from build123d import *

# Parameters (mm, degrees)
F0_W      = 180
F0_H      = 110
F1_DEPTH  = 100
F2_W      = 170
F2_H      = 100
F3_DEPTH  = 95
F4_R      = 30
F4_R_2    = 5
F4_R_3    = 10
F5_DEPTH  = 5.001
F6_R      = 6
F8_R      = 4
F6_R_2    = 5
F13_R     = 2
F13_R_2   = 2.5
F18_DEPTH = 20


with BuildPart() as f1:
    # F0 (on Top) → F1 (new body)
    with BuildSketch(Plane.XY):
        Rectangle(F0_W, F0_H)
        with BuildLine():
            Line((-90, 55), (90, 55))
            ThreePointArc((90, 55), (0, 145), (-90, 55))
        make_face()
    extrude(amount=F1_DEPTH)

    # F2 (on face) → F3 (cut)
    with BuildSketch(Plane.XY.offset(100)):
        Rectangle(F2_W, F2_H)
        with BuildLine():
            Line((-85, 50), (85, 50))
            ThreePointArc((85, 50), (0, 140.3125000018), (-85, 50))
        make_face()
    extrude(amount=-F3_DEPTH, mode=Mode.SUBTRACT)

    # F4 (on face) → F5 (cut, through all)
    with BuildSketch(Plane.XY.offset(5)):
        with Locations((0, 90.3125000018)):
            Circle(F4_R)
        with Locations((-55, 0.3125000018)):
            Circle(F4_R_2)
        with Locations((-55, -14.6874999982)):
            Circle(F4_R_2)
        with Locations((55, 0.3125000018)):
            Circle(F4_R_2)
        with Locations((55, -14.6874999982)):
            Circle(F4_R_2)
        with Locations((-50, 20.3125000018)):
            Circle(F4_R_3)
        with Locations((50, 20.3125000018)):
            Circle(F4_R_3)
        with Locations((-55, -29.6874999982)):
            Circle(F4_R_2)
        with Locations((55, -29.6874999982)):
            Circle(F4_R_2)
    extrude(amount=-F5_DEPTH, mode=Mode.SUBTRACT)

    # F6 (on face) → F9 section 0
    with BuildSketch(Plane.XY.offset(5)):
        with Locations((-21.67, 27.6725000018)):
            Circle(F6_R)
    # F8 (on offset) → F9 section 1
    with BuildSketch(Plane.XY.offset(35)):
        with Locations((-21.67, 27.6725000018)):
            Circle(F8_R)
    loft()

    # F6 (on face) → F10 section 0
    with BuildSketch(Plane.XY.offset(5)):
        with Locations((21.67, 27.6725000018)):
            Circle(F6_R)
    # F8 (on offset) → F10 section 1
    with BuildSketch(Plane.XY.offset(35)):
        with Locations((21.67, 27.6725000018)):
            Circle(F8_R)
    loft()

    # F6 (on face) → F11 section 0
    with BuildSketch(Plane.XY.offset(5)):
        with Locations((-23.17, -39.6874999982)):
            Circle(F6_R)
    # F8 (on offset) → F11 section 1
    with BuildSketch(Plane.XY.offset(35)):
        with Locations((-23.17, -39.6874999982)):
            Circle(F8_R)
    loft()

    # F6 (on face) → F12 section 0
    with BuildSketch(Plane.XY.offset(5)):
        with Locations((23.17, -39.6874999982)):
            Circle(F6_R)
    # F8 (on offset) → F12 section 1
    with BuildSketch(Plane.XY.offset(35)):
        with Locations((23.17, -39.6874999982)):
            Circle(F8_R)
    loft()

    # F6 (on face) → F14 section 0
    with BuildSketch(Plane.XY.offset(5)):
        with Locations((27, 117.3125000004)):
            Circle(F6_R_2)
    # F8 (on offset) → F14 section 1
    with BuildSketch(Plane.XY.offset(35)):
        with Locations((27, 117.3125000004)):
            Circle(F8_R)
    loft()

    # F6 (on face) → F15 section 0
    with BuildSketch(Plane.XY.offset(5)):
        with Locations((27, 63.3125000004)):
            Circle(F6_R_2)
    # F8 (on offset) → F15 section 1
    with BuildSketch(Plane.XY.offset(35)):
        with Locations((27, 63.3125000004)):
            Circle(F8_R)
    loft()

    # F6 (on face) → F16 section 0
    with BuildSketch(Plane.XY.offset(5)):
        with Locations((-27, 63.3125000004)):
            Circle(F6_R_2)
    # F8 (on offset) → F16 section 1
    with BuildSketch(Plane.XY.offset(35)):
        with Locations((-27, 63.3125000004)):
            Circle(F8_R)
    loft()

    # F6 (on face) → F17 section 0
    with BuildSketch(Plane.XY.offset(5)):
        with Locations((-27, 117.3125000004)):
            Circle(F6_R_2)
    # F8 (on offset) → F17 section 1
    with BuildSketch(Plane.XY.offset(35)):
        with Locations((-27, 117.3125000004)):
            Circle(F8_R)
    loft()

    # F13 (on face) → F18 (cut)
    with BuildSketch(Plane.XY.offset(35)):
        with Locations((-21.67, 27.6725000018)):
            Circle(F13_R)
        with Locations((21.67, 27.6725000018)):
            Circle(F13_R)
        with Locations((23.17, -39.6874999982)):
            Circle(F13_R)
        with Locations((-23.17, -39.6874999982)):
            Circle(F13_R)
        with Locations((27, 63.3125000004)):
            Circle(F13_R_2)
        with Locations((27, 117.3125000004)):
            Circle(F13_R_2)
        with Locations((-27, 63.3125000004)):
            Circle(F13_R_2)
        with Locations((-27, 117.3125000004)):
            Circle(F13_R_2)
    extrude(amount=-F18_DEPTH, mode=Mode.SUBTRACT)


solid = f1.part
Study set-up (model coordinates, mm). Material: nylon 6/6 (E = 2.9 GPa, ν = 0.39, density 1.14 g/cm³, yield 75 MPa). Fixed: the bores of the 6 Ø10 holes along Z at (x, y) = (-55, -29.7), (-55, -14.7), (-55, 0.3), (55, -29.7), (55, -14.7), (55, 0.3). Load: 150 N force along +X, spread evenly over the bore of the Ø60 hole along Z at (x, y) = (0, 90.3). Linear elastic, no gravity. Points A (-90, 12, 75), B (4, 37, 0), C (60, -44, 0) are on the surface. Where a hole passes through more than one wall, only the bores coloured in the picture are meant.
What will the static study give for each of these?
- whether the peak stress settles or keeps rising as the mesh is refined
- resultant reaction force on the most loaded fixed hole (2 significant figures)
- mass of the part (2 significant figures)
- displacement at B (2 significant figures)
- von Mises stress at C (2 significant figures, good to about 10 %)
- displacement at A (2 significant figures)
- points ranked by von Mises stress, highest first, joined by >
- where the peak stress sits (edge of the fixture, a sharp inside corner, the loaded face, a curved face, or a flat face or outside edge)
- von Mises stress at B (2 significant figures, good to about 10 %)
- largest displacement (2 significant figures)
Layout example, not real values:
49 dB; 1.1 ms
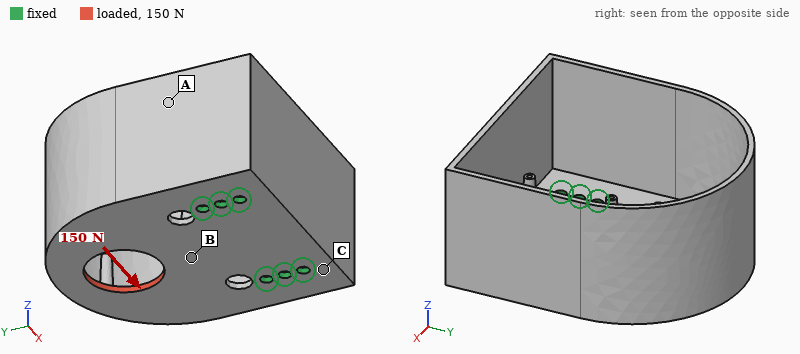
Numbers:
keeps rising; 90 N; 530 g; 13 µm; 0.20 MPa; 18 µm; B > C > A; edge of the fixture; 0.61 MPa; 49 µm
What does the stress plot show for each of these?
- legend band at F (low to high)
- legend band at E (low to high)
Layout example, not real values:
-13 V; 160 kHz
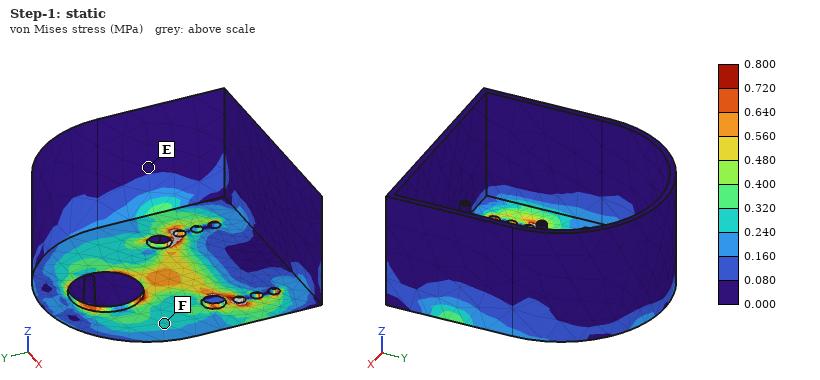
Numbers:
0.240 to 0.320 MPa; 0.000 to 0.080 MPa
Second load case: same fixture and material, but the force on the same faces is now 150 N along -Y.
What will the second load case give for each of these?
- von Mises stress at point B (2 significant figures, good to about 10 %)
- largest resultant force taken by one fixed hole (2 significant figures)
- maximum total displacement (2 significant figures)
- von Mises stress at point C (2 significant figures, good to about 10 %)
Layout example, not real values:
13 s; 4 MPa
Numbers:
0.15 MPa; 35 N; 19 µm; 0.10 MPa
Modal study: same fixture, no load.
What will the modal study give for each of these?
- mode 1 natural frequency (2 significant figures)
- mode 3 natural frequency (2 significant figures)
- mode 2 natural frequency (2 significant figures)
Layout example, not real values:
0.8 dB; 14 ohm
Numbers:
85 Hz; 190 Hz; 110 Hz
